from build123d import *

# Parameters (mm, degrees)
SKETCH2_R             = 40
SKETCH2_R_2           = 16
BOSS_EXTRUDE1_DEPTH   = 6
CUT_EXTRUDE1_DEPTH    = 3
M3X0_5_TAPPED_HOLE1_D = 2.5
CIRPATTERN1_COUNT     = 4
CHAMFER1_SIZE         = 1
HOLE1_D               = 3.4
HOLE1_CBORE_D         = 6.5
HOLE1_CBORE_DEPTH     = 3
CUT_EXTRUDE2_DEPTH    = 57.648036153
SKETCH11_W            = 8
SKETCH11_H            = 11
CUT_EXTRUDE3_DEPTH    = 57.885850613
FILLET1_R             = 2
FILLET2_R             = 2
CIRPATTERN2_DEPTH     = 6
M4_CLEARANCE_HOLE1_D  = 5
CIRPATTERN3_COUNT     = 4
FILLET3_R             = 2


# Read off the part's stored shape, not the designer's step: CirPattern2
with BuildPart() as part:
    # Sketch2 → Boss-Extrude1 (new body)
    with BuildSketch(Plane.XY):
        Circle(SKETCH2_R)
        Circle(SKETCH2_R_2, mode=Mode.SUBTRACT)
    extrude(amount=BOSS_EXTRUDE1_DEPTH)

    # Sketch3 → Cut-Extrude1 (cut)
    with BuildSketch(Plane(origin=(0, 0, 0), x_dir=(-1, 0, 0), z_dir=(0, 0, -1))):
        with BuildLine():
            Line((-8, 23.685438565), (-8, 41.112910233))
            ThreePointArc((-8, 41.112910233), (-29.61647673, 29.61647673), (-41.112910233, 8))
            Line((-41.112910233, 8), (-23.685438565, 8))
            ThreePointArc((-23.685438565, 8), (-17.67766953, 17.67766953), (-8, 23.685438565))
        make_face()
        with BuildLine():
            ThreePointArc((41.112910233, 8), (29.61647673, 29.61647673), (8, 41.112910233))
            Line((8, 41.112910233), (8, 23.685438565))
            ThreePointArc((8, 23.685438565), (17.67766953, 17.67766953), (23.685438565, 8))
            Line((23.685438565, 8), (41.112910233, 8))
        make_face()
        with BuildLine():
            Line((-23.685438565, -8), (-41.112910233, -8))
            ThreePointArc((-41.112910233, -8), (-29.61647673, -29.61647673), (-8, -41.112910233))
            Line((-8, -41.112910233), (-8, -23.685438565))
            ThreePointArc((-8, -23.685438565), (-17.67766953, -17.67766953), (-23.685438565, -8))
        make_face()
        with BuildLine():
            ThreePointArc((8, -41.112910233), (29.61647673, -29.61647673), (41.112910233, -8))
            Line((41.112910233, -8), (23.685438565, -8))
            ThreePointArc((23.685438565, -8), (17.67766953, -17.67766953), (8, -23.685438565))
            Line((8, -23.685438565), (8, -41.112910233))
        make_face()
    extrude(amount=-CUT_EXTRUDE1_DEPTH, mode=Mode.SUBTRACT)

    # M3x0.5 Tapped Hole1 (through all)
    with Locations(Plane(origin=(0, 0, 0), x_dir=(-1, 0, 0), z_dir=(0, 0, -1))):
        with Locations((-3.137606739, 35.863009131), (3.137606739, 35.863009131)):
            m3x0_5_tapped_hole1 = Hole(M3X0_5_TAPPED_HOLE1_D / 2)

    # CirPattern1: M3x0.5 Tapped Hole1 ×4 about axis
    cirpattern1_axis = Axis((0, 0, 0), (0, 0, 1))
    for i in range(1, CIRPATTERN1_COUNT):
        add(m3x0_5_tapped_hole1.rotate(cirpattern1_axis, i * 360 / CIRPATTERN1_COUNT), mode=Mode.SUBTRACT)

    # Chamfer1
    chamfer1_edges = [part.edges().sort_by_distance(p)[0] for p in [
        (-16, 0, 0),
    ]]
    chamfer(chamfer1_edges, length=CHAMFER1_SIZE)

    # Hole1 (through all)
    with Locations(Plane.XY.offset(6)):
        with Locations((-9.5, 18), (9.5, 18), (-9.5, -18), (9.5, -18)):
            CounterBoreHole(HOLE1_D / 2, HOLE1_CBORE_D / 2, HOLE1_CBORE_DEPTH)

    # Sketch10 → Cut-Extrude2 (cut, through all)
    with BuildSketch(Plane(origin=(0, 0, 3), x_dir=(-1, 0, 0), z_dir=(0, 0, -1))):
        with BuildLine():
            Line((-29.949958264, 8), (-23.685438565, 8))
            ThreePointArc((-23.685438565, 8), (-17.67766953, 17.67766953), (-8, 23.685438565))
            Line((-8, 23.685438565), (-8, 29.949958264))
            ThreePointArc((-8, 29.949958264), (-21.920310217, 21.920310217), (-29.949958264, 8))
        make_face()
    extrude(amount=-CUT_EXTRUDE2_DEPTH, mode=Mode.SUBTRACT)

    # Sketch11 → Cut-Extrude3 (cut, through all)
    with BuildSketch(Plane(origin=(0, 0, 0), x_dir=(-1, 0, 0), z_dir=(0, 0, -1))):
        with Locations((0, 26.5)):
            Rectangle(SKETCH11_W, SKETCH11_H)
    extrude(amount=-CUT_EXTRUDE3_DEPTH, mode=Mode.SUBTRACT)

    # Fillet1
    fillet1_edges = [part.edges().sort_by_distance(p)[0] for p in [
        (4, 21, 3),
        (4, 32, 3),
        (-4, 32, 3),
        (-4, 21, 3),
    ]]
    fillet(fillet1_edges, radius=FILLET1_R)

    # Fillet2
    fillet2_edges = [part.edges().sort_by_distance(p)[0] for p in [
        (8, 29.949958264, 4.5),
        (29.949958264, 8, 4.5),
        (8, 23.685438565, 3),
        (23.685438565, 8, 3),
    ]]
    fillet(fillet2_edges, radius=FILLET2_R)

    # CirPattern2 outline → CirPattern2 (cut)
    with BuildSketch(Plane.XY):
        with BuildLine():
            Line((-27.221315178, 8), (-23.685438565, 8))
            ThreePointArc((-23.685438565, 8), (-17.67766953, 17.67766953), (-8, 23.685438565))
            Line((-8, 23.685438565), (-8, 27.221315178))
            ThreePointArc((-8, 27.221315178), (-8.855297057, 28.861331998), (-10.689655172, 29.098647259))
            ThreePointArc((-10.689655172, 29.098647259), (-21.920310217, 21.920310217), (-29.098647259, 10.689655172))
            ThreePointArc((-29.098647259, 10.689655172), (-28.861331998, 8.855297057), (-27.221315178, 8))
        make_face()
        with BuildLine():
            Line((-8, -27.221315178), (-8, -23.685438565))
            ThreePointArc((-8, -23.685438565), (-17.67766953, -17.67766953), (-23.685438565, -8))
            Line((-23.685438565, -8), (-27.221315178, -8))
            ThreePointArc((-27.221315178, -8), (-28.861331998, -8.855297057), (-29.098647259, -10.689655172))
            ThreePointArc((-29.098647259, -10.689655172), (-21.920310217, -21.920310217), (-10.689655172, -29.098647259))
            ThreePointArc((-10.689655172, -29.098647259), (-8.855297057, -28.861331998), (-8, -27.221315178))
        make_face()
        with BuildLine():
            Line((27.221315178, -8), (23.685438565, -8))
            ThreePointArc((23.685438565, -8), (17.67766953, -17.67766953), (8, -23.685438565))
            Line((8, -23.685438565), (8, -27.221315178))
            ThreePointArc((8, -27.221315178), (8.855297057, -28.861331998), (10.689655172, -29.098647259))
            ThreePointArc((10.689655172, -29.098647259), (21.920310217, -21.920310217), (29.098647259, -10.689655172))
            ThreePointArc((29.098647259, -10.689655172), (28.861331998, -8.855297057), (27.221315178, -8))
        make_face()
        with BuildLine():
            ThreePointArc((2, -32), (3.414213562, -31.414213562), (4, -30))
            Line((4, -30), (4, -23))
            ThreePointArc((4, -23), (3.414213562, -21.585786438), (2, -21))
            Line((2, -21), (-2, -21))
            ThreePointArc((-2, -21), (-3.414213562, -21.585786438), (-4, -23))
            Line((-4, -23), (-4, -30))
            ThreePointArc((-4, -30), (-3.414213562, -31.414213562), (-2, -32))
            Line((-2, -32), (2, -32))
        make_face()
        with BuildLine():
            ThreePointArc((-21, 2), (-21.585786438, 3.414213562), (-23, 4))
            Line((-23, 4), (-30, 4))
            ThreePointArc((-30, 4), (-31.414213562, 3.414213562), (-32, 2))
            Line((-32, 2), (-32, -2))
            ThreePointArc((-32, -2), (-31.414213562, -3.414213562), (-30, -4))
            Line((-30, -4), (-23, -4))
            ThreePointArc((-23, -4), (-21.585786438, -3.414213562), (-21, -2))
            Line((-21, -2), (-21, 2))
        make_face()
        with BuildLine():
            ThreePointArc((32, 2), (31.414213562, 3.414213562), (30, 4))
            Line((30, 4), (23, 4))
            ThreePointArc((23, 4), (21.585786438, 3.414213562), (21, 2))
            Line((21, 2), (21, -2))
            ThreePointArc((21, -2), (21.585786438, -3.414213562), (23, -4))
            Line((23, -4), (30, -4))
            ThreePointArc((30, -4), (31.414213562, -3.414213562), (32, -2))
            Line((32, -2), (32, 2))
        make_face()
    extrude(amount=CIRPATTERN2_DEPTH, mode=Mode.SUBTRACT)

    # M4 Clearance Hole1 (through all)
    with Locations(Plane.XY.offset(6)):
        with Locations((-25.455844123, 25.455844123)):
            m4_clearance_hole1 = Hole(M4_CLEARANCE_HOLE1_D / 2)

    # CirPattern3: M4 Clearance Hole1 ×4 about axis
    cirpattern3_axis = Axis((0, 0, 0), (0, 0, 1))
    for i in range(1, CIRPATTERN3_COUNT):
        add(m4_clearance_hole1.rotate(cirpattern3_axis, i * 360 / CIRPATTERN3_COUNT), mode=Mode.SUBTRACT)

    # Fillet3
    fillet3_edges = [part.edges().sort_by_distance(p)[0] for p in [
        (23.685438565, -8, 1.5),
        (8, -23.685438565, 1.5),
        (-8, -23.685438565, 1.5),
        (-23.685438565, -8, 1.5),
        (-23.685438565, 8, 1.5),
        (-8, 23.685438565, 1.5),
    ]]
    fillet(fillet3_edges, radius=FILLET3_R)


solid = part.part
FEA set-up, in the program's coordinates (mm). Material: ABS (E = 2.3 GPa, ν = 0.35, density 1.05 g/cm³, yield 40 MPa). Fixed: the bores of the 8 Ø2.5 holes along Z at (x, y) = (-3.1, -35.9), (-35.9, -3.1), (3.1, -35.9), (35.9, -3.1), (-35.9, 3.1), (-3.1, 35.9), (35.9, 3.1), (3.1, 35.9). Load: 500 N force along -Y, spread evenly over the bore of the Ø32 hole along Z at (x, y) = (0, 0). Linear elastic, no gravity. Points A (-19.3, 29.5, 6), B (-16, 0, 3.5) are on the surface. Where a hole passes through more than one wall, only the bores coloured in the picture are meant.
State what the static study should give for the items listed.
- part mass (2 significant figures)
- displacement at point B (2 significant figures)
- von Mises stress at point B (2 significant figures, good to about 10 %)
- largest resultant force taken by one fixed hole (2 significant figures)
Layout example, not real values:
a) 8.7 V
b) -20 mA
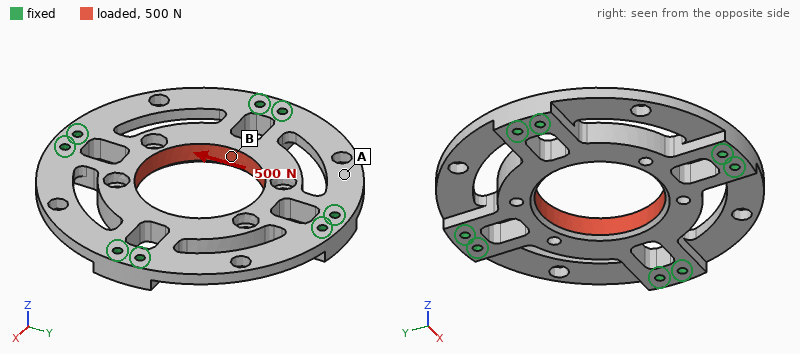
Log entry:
a) 15 g
b) 69 µm
c) 2.0 MPa
d) 92 N
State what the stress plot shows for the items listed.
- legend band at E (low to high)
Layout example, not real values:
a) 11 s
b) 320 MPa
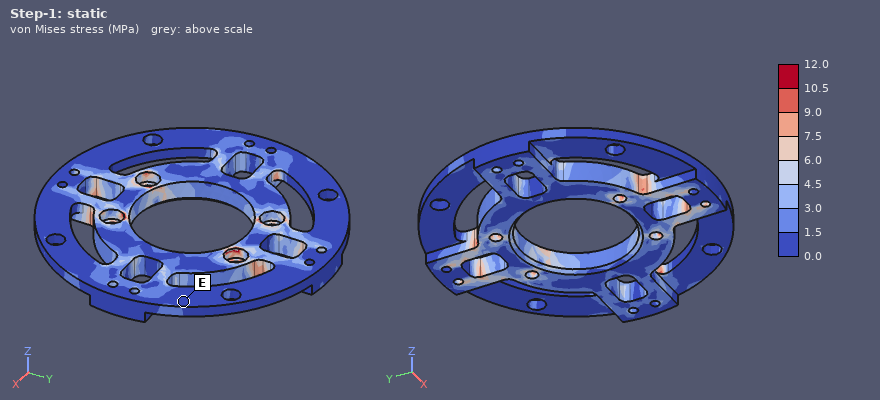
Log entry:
a) 0.0 to 1.5 MPa
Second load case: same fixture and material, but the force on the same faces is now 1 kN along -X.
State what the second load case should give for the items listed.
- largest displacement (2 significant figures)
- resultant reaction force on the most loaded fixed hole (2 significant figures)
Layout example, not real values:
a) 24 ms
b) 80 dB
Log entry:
a) 0.12 mm
b) 190 N
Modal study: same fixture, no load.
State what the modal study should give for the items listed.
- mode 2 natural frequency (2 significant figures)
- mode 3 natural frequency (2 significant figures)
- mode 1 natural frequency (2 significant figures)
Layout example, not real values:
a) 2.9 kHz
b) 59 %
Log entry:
a) 2300 Hz
b) 2300 Hz
c) 2300 Hz
